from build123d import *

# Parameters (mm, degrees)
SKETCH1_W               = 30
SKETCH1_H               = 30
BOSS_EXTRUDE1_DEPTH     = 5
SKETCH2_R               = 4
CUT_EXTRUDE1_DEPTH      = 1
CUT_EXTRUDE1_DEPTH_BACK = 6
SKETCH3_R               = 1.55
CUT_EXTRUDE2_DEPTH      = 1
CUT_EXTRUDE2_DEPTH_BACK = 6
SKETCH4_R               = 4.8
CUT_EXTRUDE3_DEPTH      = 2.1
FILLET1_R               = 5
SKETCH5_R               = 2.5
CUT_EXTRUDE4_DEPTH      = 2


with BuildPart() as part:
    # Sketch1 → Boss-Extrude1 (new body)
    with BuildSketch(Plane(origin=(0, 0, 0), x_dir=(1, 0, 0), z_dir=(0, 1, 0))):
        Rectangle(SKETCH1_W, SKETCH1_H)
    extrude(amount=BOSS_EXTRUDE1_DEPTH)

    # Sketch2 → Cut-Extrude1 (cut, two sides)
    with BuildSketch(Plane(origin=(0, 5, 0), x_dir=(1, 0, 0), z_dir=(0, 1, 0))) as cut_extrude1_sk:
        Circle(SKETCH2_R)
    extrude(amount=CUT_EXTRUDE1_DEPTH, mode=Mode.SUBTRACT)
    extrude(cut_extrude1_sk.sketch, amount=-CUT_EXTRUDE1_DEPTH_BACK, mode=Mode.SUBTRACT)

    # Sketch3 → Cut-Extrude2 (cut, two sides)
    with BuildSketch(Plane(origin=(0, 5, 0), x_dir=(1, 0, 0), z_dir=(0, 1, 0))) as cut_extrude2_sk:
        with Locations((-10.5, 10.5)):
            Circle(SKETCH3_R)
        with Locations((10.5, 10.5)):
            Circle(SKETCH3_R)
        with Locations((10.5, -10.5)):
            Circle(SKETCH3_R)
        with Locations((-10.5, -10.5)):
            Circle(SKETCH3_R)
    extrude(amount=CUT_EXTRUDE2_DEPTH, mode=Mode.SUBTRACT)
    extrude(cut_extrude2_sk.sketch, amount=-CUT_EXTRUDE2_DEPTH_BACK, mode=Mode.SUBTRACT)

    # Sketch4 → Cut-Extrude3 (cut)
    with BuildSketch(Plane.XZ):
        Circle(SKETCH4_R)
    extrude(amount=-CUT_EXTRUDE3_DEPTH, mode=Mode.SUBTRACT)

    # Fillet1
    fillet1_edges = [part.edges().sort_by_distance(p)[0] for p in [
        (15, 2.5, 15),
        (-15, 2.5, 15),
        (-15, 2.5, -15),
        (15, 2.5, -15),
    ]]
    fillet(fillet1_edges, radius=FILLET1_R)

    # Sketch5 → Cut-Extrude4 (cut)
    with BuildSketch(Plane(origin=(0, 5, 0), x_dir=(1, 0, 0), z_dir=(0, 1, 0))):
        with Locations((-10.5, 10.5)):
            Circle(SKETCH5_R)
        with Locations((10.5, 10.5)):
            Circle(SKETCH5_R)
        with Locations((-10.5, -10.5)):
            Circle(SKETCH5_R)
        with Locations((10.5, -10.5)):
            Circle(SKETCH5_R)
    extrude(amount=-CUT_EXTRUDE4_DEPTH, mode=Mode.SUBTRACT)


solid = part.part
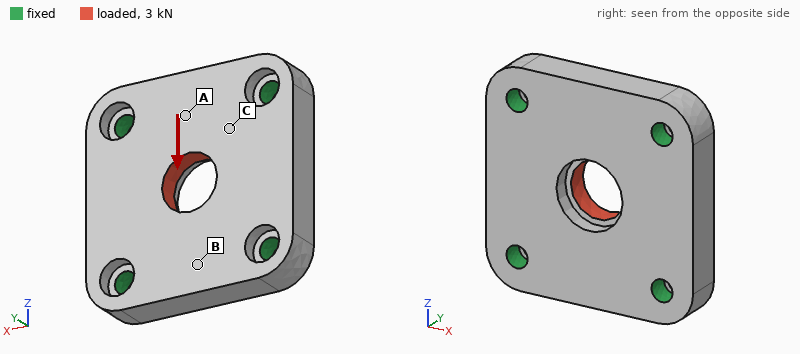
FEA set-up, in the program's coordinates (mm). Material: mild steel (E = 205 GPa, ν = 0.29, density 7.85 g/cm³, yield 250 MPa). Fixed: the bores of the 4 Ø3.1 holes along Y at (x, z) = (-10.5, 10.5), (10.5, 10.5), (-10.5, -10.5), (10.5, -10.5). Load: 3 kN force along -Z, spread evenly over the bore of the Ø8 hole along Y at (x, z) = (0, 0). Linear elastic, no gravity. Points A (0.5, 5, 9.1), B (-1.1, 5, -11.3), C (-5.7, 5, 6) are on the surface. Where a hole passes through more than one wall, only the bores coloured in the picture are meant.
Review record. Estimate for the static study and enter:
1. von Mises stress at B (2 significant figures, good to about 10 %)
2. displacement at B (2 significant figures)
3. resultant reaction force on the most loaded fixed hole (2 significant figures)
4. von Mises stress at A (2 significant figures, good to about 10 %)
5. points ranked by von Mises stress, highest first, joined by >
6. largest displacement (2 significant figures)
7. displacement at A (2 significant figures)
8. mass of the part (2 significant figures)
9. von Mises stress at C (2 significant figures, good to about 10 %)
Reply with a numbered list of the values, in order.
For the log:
1. 8.2 MPa
2. 1.5 µm
3. 810 N
4. 15 MPa
5. C > A > B
6. 2.5 µm
7. 1.6 µm
8. 30 g
9. 27 MPa
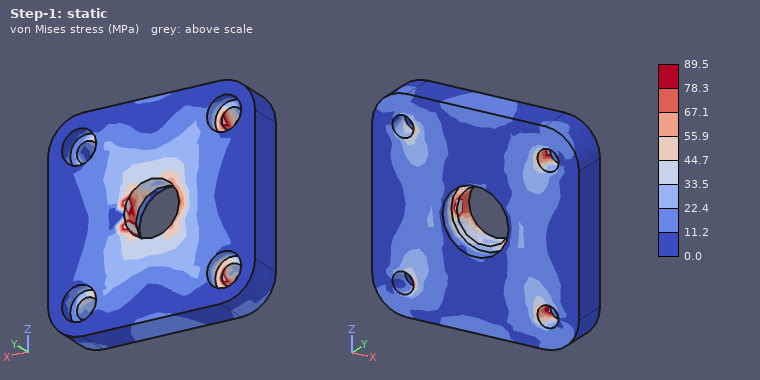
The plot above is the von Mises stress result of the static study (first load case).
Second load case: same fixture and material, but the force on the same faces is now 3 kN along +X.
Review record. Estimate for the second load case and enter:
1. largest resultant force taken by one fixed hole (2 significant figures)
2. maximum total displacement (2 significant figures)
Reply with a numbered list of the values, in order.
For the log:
1. 810 N
2. 2.5 µm
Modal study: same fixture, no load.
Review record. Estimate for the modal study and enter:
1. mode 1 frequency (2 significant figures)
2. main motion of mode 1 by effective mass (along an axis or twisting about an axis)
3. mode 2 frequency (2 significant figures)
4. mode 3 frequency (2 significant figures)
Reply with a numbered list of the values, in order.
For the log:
1. 32 kHz
2. along Y
3. 41 kHz
4. 42 kHz
